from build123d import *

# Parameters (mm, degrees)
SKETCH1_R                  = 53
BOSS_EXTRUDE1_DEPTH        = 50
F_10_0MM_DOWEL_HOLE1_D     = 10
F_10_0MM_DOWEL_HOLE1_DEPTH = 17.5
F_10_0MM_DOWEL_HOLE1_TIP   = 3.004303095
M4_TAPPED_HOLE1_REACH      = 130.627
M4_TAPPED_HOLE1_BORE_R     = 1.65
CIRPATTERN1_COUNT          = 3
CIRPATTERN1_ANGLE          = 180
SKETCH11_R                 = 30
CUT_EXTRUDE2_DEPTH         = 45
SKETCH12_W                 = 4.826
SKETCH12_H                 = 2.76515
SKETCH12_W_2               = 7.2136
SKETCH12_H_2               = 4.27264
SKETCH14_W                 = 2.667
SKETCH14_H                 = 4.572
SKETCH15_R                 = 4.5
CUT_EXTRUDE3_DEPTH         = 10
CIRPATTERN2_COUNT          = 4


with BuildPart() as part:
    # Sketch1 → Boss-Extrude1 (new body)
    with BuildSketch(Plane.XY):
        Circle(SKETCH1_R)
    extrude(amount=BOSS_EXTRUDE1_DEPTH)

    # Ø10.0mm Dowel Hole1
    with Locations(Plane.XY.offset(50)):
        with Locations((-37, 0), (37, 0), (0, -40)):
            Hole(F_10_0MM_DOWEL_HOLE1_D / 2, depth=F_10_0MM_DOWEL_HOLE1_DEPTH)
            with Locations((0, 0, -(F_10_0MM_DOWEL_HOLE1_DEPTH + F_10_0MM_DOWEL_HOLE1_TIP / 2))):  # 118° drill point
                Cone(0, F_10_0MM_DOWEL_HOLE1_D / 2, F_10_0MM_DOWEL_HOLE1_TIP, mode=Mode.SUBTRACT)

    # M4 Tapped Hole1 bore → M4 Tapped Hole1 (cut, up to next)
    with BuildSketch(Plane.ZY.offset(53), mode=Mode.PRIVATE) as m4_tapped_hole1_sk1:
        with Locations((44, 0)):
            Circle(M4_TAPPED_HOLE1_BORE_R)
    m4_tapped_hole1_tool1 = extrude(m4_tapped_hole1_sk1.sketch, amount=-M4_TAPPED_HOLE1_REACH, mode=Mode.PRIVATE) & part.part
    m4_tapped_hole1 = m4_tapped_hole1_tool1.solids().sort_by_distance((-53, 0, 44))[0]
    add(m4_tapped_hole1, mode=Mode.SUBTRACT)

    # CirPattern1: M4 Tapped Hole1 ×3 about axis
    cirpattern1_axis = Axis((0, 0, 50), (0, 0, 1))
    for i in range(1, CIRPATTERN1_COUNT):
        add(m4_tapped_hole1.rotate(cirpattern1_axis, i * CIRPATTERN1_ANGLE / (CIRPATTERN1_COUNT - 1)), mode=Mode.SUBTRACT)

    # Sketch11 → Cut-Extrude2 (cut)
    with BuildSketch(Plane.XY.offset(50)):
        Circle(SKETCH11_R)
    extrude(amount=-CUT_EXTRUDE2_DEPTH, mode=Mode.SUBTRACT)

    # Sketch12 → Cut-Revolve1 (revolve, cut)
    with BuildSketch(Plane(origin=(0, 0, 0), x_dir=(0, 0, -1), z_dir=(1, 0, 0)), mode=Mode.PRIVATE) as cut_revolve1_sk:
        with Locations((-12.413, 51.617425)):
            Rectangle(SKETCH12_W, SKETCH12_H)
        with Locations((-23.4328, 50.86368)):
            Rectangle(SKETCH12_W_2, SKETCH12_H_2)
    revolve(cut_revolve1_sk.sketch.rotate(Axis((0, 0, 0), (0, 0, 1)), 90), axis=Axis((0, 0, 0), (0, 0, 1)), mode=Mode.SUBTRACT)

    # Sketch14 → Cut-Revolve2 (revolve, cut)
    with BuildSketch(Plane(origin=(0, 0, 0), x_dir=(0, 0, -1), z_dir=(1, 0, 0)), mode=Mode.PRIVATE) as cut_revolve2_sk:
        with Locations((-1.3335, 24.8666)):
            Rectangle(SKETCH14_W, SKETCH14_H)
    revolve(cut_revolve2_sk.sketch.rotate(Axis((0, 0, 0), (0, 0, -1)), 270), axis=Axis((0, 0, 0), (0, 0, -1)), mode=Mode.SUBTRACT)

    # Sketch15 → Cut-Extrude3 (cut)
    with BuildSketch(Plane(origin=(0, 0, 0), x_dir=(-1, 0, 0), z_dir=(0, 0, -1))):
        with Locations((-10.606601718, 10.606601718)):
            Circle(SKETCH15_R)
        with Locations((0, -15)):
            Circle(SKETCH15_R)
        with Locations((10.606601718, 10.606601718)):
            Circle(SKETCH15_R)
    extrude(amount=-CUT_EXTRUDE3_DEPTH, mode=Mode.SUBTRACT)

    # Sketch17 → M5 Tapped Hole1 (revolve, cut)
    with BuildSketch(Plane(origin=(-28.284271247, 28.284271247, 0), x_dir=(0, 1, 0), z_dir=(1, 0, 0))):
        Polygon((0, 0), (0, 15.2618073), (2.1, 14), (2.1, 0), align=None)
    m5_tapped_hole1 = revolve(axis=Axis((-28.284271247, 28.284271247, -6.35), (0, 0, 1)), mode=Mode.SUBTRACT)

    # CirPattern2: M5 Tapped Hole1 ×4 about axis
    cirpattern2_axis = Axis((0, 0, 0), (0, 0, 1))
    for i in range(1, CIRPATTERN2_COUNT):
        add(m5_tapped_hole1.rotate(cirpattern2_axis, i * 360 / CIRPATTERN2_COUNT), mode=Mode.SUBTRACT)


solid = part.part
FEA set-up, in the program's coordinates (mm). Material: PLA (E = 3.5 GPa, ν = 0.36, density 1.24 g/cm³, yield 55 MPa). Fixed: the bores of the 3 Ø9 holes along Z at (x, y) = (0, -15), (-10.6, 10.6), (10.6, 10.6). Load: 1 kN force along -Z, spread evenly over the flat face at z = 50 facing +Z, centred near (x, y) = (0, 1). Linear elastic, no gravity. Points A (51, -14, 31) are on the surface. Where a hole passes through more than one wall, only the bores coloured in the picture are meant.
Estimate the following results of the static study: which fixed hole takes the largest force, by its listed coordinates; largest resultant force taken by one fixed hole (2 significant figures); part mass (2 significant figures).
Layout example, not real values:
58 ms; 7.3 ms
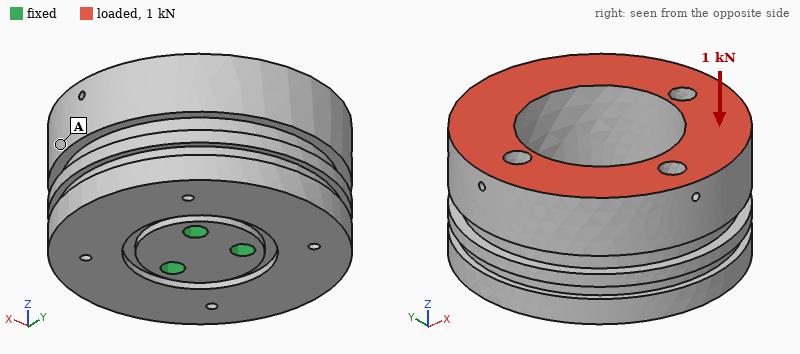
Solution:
(0, -15); 400 N; 360 g
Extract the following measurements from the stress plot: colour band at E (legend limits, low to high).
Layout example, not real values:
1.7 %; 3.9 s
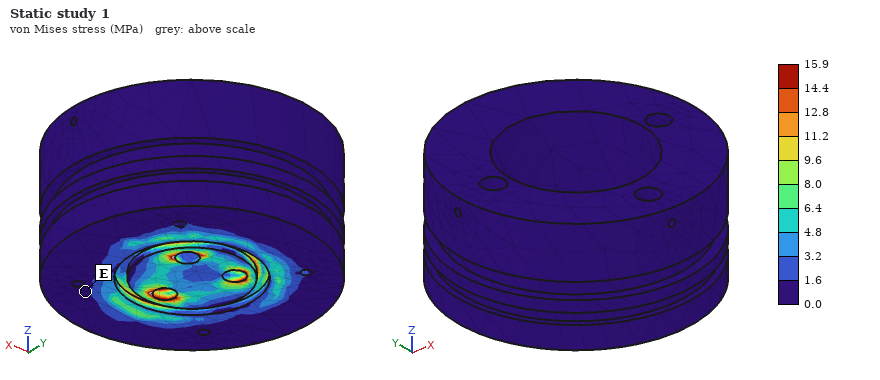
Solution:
0.0 to 1.6 MPa
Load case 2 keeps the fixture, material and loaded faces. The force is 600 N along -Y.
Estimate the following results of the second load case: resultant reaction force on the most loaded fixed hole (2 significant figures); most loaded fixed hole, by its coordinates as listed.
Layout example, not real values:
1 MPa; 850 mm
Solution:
720 N; (0, -15)
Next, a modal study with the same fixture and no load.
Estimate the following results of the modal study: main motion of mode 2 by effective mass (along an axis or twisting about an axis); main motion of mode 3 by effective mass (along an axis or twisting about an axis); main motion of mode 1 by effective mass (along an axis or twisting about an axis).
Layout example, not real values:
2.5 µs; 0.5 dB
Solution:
along Y; along Z; along X
